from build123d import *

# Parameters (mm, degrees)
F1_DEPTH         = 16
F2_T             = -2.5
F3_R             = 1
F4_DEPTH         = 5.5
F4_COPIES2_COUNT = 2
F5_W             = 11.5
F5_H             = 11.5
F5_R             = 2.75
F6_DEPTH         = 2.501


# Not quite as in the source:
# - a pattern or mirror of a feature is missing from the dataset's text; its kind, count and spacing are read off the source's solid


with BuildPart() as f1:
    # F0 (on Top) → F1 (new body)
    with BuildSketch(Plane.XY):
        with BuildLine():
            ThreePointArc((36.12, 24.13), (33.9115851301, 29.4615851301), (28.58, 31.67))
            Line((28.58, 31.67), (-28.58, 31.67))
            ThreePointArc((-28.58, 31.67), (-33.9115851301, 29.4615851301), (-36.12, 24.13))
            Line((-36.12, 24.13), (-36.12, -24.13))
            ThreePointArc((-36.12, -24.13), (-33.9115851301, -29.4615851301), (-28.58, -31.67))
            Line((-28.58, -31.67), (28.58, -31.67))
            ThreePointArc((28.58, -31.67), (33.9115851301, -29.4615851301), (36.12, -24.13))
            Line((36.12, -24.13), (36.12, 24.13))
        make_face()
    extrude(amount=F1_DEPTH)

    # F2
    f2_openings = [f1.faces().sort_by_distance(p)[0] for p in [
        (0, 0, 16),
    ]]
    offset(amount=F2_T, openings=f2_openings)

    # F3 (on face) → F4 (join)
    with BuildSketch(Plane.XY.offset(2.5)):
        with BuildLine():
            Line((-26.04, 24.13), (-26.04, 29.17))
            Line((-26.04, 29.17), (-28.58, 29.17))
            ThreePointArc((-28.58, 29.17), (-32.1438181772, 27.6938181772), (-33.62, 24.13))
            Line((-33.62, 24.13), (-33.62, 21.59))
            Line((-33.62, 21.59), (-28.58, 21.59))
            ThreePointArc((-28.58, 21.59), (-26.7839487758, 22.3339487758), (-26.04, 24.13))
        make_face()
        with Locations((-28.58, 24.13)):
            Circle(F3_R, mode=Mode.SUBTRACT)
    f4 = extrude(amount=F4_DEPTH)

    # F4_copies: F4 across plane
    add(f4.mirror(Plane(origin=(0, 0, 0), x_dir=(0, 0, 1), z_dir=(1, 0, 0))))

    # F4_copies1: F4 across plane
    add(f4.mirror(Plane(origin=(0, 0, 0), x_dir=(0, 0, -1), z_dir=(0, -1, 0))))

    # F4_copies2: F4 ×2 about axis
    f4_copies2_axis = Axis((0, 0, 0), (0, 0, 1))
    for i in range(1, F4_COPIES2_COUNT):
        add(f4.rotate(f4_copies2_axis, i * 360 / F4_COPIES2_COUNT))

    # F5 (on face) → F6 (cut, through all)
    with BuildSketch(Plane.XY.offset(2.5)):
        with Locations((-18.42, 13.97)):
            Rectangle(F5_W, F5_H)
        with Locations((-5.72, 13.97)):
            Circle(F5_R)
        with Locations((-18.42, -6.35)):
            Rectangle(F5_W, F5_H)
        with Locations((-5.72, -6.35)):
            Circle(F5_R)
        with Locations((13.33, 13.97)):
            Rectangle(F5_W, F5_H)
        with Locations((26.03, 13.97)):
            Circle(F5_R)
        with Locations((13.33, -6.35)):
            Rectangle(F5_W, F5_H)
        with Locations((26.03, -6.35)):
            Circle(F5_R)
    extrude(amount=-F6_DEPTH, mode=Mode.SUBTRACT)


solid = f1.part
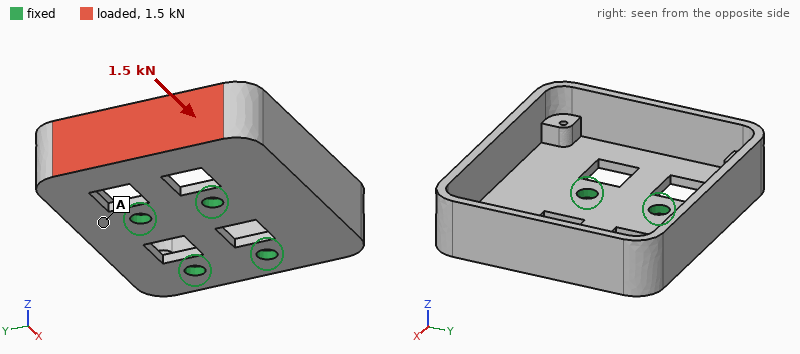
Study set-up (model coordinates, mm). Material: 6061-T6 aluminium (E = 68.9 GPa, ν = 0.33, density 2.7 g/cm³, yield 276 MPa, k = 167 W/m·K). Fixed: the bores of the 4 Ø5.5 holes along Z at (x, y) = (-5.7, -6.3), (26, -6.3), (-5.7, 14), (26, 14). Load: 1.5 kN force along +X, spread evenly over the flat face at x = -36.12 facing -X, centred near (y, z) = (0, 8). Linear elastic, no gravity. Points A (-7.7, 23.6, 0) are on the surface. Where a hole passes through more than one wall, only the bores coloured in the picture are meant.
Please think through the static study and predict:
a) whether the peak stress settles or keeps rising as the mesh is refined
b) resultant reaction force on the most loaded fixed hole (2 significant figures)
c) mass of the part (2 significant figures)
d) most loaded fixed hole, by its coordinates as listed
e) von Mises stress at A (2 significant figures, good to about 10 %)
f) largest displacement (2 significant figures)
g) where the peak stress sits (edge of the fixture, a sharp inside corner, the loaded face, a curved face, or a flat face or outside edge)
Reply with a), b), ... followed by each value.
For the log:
a) keeps rising
b) 790 N
c) 52 g
d) (-5.7, -6.3)
e) 18 MPa
f) 0.30 mm
g) a sharp inside corner
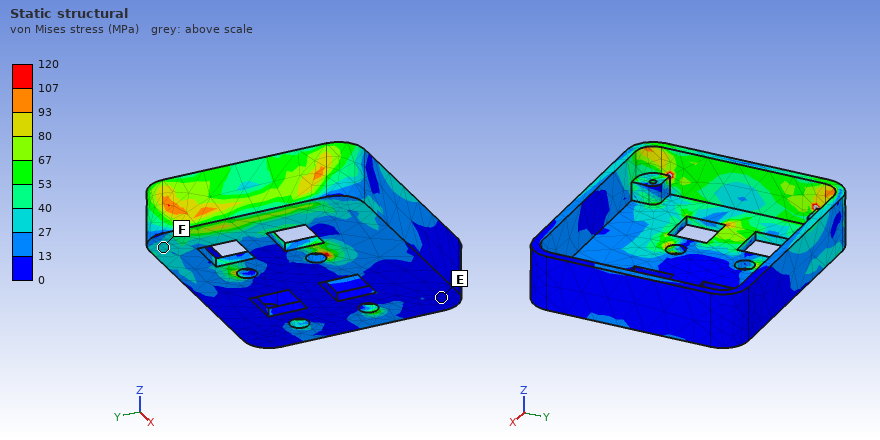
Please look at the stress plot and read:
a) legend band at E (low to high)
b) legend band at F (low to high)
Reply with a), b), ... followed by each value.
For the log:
a) 0 to 13 MPa
b) 27 to 40 MPa
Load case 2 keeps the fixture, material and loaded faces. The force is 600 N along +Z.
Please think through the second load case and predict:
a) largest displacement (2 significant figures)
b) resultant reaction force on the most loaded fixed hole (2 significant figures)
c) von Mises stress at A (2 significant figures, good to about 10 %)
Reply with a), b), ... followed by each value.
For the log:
a) 0.45 mm
b) 530 N
c) 59 MPa
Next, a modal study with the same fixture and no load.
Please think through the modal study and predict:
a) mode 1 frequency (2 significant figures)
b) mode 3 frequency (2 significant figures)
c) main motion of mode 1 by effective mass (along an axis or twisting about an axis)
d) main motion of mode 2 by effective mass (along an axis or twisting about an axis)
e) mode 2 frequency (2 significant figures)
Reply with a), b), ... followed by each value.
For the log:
a) 1500 Hz
b) 4000 Hz
c) along Z
d) along Z
e) 2200 Hz
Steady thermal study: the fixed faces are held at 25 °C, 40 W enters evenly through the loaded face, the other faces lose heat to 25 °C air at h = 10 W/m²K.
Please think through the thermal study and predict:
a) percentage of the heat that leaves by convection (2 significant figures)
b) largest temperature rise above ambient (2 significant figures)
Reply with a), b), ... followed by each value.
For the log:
a) 6.8 %
b) 64 K
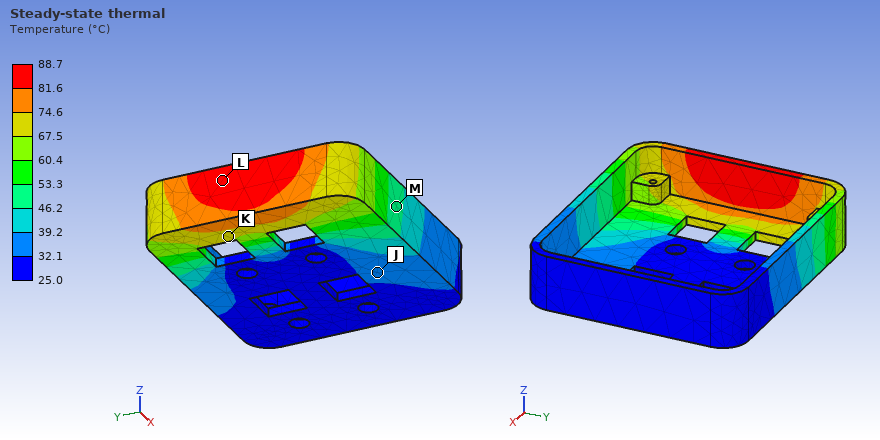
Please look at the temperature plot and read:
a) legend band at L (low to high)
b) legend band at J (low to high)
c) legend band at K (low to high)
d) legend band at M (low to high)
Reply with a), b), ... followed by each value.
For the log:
a) 81.6 to 88.7 °C
b) 32.1 to 39.2 °C
c) 67.5 to 74.6 °C
d) 46.2 to 53.3 °C
